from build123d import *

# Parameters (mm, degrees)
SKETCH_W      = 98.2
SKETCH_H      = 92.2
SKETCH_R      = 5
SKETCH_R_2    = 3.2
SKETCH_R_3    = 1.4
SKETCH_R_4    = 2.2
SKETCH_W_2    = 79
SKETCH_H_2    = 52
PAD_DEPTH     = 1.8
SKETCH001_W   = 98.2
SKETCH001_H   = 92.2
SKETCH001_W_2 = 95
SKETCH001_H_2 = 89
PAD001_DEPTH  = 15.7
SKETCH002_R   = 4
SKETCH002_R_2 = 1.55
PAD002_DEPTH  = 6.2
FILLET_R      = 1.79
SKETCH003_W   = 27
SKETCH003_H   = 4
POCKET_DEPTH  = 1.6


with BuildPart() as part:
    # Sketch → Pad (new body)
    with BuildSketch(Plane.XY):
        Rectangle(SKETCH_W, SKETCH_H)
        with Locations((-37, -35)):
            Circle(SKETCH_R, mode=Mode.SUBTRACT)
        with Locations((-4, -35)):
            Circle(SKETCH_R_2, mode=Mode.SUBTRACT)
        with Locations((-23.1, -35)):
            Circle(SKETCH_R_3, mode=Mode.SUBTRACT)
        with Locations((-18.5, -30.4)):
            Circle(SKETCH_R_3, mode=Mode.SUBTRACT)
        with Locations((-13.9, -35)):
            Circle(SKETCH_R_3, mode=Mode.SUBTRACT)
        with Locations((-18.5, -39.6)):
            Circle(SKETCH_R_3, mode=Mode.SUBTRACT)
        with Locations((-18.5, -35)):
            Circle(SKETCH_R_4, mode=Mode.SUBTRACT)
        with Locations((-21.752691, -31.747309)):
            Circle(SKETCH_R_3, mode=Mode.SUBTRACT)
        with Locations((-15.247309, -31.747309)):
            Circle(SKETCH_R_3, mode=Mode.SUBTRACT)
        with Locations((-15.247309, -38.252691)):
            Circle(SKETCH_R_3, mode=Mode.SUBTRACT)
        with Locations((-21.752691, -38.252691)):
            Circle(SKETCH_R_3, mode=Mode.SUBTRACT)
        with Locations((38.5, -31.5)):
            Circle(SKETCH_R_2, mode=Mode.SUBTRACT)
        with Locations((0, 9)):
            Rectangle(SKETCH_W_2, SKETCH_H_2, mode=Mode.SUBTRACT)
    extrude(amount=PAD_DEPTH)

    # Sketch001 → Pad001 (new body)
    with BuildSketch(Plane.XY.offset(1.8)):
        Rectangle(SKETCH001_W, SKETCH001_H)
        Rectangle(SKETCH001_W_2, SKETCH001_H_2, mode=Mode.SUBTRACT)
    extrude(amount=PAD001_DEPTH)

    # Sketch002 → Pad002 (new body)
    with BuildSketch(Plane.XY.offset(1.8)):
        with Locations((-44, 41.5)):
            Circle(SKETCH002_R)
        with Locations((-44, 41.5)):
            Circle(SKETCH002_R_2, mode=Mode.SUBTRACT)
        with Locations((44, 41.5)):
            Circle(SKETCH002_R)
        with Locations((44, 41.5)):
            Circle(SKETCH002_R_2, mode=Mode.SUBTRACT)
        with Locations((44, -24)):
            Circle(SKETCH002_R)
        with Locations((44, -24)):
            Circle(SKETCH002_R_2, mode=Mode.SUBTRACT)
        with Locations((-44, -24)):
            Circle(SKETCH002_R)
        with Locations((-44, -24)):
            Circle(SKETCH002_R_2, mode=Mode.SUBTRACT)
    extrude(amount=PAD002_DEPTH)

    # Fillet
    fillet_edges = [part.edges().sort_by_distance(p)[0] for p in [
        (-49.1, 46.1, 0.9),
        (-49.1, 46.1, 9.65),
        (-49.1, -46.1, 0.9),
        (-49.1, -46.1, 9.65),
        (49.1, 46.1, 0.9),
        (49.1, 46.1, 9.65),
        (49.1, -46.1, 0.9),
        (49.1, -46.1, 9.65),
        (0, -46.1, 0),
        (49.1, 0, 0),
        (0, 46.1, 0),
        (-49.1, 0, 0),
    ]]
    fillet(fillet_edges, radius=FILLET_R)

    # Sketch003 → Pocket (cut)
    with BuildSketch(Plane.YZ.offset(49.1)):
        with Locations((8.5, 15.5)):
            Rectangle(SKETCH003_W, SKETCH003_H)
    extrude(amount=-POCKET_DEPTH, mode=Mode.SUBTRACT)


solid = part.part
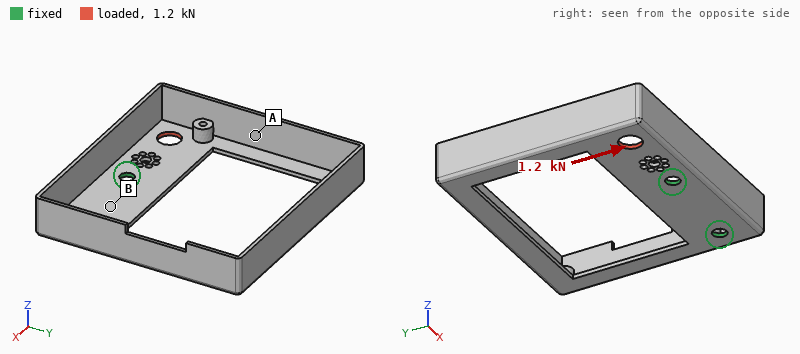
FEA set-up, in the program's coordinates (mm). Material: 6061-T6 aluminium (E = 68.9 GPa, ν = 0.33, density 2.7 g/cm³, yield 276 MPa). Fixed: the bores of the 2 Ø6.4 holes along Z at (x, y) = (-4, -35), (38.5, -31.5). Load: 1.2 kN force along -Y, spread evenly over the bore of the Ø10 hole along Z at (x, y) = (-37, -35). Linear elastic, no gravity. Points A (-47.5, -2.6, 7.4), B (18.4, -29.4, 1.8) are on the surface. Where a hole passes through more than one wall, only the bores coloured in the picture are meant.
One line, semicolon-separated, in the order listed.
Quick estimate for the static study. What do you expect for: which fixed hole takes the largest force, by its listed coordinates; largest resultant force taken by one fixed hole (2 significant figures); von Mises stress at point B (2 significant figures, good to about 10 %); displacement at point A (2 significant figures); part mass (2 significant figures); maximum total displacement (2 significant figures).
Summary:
(-4, -35); 1.9 kN; 33 MPa; 0.25 mm; 50 g; 0.29 mm
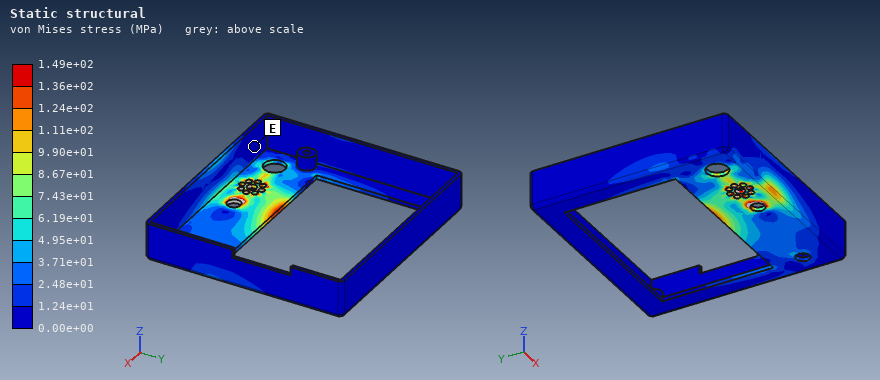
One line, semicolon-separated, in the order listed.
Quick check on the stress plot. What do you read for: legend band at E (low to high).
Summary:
0.00e+00 to 1.24e+01 MPa
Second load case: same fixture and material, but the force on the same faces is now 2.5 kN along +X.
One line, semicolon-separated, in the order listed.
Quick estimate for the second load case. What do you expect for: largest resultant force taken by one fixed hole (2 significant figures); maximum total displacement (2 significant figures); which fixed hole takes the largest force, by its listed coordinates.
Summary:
2.1 kN; 0.10 mm; (-4, -35)
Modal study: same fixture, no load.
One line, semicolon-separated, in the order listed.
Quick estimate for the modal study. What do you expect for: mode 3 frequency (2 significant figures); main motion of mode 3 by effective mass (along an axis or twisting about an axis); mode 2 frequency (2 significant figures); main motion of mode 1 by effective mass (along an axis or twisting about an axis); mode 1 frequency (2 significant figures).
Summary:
1000 Hz; along X; 510 Hz; along Z; 200 Hz
